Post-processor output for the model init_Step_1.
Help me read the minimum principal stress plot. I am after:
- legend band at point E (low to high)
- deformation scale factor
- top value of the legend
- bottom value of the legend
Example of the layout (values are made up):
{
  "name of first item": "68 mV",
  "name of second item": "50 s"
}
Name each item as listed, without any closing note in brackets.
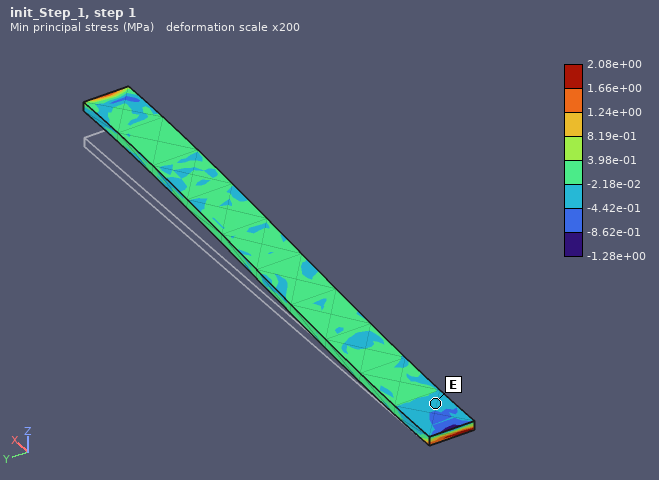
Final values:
{
  "legend band at point E": "-4.42e-01 to -2.18e-02 MPa",
  "deformation scale factor": "200",
  "top value of the legend": "2.08e+00 MPa",
  "bottom value of the legend": "-1.28e+00 MPa"
}
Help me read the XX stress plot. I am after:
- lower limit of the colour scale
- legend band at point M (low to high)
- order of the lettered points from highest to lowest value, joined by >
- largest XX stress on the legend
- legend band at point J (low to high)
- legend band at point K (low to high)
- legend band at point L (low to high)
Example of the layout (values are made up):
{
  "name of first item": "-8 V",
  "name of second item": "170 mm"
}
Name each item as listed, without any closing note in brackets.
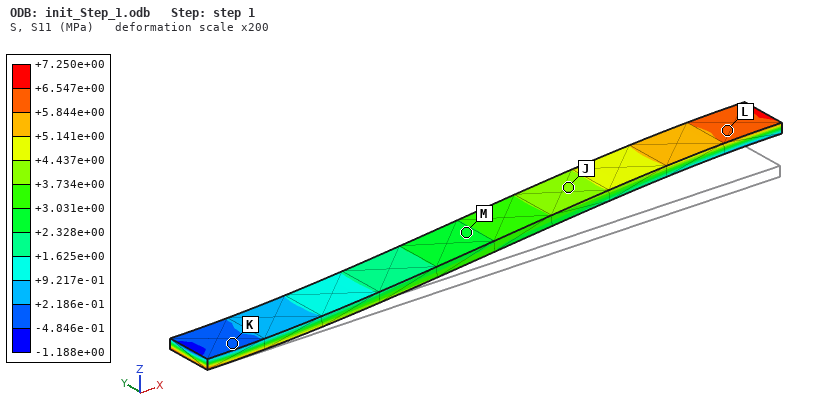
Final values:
{
  "lower limit of the colour scale": "-1.188e+00 MPa",
  "legend band at point M": "+2.328e+00 to +3.031e+00 MPa",
  "order of the lettered points from highest to lowest value, joined by >": "L > J > M > K",
  "largest XX stress on the legend": "+7.250e+00 MPa",
  "legend band at point J": "+3.734e+00 to +4.437e+00 MPa",
  "legend band at point K": "-4.846e-01 to +2.186e-01 MPa",
  "legend band at point L": "+5.844e+00 to +6.547e+00 MPa"
}
